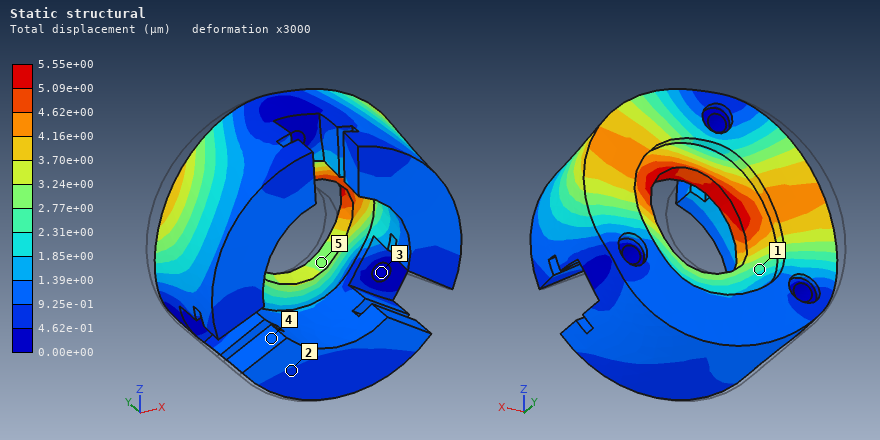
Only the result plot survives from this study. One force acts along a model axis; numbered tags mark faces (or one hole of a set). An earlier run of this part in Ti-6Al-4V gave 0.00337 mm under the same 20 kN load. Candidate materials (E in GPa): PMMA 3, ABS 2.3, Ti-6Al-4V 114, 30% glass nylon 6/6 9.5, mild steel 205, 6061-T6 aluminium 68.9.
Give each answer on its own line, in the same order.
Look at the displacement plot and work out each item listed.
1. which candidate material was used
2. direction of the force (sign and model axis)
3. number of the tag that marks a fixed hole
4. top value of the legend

6061-T6 aluminium
+X
3
5.55e+00 µm
